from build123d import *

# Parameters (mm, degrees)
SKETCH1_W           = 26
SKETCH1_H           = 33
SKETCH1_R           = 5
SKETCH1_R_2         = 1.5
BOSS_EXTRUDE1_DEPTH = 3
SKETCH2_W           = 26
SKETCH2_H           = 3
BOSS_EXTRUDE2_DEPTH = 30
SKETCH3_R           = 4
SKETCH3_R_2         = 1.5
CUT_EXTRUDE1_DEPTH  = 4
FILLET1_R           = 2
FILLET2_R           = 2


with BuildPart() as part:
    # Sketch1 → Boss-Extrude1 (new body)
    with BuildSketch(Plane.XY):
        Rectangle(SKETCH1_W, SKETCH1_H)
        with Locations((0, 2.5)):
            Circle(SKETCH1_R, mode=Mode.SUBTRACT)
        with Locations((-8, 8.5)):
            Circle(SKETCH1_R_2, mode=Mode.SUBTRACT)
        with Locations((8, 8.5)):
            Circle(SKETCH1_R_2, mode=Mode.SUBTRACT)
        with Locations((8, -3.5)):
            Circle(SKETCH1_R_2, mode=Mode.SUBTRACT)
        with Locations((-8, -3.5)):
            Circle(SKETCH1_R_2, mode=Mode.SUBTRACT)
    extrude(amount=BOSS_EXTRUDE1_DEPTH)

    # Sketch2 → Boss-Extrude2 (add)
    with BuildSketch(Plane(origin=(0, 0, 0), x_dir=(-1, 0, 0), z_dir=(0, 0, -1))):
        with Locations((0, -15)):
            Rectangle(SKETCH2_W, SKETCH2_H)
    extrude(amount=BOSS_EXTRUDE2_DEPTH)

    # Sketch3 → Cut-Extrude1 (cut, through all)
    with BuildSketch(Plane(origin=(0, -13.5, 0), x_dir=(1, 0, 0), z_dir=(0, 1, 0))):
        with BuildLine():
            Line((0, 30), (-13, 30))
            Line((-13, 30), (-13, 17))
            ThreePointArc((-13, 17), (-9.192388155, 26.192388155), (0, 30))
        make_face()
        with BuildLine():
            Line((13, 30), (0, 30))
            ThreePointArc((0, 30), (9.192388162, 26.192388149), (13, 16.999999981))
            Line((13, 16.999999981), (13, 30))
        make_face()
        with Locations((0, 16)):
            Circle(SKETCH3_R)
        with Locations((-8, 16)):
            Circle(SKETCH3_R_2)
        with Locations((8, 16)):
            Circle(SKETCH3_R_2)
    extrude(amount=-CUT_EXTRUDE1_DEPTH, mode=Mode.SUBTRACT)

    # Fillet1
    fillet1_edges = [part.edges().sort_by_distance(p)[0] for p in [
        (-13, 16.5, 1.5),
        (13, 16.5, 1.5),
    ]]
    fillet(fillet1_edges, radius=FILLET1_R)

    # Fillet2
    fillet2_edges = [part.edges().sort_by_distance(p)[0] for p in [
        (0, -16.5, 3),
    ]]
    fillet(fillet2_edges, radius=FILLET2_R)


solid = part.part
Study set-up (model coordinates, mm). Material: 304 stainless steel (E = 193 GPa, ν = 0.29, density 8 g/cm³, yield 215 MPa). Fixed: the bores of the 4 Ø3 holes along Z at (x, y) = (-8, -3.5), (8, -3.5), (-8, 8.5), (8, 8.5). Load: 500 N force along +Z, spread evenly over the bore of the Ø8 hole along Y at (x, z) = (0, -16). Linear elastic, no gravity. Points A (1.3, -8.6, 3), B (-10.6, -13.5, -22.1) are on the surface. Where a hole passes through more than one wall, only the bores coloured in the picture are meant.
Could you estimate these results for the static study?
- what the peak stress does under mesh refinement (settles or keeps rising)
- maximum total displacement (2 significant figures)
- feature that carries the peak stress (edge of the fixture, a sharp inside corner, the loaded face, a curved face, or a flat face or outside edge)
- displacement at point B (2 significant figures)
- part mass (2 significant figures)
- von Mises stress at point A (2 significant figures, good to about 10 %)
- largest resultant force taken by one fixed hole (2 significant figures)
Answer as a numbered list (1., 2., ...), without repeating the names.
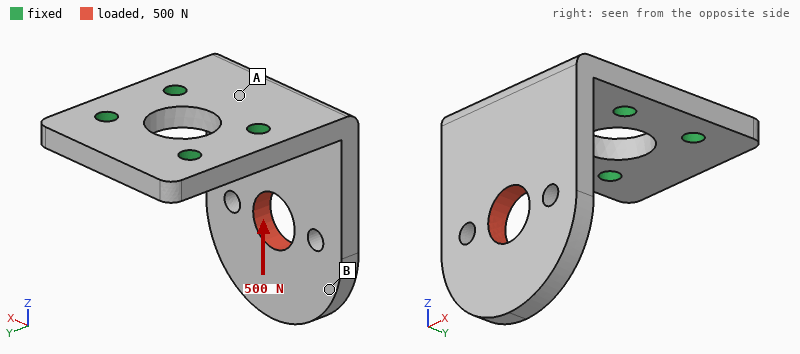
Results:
1. keeps rising
2. 95 µm
3. edge of the fixture
4. 71 µm
5. 33 g
6. 61 MPa
7. 280 N
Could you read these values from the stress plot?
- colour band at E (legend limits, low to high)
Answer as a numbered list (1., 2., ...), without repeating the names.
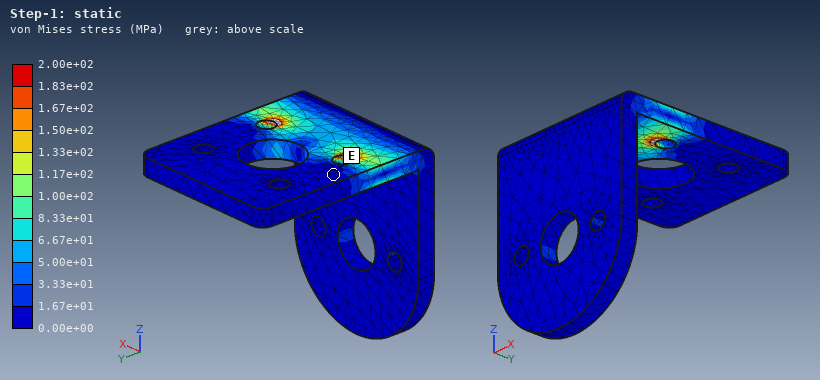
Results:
1. 0.00e+00 to 1.67e+01 MPa
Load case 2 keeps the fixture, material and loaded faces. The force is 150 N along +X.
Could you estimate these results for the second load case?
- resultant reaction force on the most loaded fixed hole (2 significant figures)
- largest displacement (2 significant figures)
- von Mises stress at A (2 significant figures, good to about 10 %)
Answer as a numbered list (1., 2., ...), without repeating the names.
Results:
1. 190 N
2. 22 µm
3. 19 MPa
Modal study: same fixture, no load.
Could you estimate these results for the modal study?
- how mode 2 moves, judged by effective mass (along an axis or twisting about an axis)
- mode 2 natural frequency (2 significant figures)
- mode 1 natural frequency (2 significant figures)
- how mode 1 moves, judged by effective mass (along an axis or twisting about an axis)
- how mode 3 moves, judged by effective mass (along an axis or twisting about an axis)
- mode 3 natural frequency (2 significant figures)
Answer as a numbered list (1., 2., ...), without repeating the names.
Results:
1. along X
2. 4100 Hz
3. 1800 Hz
4. along Y
5. along Z
6. 7100 Hz
